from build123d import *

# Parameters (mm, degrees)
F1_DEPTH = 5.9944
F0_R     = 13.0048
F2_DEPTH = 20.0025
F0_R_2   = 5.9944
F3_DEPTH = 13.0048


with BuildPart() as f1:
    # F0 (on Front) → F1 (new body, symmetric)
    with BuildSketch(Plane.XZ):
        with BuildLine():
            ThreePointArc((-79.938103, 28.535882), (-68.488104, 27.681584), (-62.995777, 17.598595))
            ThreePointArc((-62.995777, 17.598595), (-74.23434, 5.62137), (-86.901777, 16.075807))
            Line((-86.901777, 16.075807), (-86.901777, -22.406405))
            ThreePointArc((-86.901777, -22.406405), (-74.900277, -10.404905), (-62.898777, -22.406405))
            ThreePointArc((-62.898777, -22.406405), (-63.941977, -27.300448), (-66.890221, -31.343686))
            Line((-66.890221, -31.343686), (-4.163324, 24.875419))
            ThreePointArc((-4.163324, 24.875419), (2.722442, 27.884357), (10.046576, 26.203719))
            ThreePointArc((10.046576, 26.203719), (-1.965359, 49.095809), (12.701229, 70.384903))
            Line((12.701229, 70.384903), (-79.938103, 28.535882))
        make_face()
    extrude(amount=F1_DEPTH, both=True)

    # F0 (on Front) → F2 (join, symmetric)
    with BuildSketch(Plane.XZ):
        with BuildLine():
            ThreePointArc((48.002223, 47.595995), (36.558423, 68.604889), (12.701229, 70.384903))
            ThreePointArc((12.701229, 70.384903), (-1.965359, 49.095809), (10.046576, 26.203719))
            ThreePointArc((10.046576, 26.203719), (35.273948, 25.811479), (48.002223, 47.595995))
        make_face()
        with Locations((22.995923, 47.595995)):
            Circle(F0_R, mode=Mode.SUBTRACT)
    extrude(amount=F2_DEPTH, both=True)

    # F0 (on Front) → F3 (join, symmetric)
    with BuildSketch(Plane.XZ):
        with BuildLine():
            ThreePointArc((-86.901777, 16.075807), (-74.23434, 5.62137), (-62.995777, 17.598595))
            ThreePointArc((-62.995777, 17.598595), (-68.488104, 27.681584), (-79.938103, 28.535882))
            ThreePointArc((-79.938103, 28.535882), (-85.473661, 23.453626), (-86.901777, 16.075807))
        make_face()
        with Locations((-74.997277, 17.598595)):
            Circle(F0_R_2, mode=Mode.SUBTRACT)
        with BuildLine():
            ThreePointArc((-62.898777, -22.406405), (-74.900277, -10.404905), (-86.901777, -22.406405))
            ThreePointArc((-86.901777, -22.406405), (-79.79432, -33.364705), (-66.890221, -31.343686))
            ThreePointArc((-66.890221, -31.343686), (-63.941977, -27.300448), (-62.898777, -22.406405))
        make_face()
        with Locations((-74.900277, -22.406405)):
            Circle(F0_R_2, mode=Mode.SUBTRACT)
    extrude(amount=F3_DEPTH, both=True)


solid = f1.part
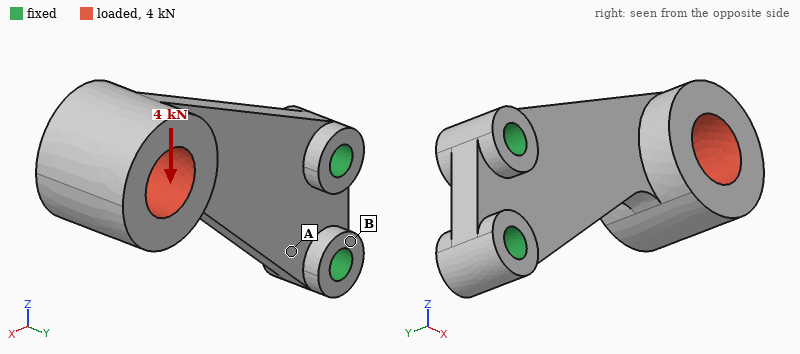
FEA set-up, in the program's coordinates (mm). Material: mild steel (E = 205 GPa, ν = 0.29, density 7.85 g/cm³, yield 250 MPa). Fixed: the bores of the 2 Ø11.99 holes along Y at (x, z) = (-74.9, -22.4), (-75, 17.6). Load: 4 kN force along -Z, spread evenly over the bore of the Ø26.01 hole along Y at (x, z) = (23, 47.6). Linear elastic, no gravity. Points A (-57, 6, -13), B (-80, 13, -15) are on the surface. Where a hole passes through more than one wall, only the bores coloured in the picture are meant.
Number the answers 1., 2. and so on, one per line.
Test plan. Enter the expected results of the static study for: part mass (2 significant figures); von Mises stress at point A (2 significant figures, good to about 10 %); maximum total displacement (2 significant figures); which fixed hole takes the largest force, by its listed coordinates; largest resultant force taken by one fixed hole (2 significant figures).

1. 940 g
2. 44 MPa
3. 0.11 mm
4. (-74.9, -22.4)
5. 9.5 kN
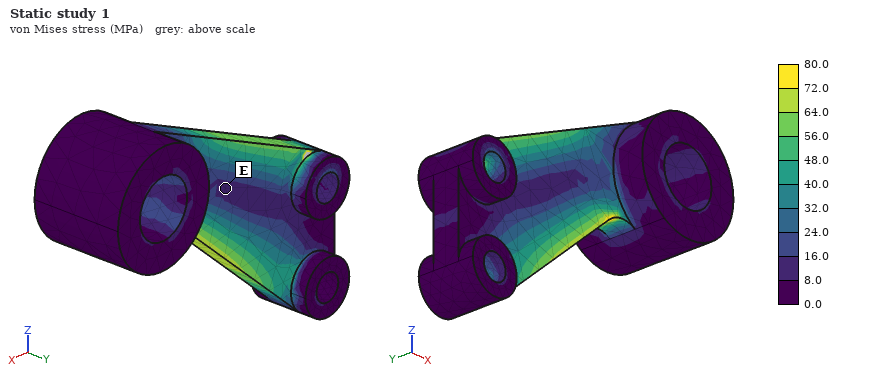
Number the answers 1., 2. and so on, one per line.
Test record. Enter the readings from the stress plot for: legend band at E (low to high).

1. 8.0 to 16.0 MPa
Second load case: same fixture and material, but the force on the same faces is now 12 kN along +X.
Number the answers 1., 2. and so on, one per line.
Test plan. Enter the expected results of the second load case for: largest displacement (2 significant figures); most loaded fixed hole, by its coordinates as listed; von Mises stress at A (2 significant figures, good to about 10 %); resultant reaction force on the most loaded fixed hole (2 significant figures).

1. 0.12 mm
2. (-75, 17.6)
3. 40 MPa
4. 19 kN
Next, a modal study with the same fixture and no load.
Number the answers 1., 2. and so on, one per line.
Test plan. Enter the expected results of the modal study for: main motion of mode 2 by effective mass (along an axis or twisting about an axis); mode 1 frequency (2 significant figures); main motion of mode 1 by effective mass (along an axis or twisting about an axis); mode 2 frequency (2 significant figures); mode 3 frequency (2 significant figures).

1. along Z
2. 460 Hz
3. along Y
4. 1500 Hz
5. 1900 Hz
